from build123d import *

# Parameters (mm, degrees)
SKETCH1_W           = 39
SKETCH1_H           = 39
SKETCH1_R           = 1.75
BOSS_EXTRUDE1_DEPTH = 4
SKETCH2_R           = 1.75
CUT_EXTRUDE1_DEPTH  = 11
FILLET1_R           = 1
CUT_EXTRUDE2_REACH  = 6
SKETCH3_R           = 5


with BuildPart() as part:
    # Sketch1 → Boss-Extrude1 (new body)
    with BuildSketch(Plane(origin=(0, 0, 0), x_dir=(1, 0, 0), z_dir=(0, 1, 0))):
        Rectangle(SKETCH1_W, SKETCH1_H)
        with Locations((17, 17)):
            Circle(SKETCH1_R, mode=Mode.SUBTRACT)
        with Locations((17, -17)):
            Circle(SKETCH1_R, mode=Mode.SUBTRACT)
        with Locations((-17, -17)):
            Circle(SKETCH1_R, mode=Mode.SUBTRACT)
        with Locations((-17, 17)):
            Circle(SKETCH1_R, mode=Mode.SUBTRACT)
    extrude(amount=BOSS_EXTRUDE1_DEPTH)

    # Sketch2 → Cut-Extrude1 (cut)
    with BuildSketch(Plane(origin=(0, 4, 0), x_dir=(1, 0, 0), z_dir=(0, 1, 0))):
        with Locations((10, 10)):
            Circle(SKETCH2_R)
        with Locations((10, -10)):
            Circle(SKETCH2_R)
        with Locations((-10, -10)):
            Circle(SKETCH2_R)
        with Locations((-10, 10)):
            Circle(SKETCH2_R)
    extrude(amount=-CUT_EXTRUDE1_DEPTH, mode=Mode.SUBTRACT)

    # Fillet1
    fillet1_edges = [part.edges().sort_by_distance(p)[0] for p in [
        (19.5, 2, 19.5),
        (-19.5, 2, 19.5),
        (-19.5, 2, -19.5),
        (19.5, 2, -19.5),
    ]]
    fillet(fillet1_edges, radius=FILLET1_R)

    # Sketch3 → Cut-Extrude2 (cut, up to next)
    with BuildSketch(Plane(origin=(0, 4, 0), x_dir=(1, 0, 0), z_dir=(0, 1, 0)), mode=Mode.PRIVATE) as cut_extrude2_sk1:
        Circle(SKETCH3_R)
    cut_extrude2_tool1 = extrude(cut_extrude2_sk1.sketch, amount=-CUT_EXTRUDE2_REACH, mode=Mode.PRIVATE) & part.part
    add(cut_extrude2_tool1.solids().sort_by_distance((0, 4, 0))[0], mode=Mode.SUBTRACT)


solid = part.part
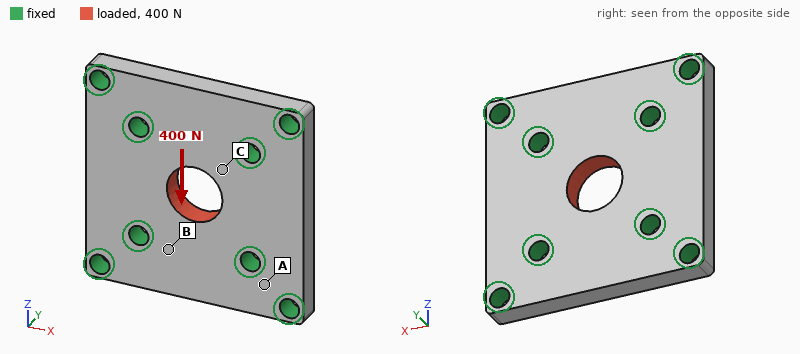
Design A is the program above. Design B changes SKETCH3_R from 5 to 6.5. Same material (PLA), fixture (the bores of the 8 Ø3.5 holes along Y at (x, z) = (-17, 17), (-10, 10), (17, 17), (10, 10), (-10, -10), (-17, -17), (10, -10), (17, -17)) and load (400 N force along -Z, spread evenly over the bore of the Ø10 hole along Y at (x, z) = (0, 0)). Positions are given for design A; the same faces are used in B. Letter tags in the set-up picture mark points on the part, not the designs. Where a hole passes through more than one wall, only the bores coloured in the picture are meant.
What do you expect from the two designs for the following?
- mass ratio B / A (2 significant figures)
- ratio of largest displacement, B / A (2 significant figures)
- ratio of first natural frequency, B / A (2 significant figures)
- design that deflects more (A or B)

0.96
0.89
1.00
A
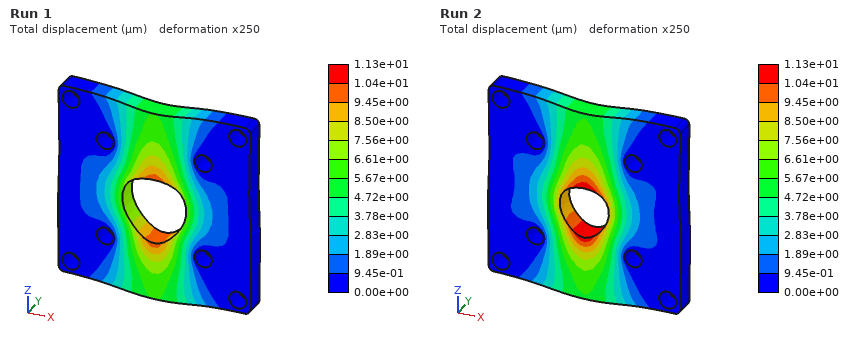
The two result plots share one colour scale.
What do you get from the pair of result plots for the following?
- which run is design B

Run 1
